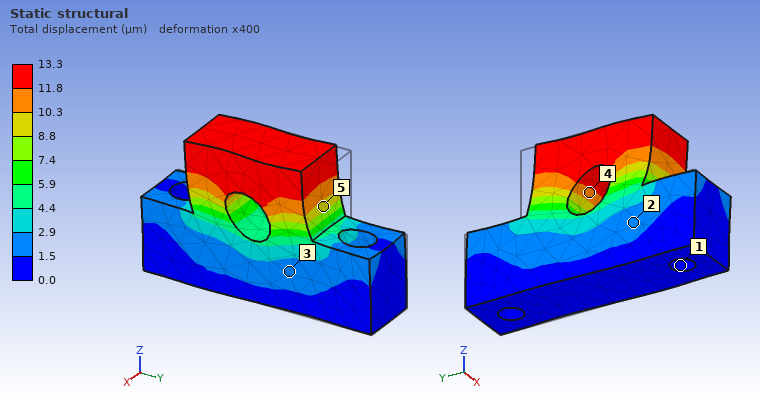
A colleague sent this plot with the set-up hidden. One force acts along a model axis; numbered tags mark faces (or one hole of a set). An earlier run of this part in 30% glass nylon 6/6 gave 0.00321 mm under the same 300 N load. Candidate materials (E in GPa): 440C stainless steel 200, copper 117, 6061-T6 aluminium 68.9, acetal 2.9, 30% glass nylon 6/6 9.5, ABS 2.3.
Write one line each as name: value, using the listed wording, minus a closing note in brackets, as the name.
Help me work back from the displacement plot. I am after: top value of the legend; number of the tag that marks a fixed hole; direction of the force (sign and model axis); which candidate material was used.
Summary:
top value of the legend: 13.3 µm
number of the tag that marks a fixed hole: 1
direction of the force: -Y
which candidate material was used: ABS
